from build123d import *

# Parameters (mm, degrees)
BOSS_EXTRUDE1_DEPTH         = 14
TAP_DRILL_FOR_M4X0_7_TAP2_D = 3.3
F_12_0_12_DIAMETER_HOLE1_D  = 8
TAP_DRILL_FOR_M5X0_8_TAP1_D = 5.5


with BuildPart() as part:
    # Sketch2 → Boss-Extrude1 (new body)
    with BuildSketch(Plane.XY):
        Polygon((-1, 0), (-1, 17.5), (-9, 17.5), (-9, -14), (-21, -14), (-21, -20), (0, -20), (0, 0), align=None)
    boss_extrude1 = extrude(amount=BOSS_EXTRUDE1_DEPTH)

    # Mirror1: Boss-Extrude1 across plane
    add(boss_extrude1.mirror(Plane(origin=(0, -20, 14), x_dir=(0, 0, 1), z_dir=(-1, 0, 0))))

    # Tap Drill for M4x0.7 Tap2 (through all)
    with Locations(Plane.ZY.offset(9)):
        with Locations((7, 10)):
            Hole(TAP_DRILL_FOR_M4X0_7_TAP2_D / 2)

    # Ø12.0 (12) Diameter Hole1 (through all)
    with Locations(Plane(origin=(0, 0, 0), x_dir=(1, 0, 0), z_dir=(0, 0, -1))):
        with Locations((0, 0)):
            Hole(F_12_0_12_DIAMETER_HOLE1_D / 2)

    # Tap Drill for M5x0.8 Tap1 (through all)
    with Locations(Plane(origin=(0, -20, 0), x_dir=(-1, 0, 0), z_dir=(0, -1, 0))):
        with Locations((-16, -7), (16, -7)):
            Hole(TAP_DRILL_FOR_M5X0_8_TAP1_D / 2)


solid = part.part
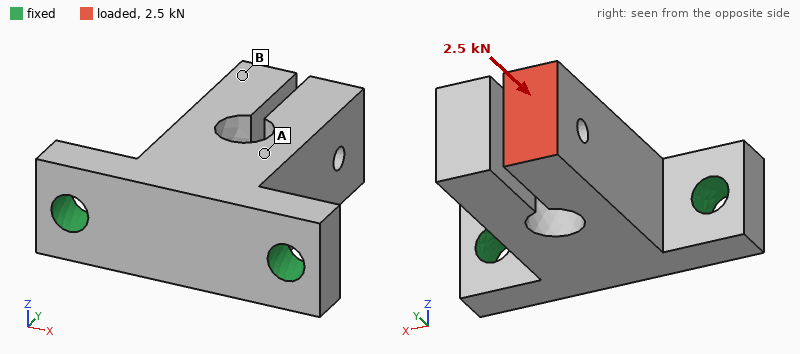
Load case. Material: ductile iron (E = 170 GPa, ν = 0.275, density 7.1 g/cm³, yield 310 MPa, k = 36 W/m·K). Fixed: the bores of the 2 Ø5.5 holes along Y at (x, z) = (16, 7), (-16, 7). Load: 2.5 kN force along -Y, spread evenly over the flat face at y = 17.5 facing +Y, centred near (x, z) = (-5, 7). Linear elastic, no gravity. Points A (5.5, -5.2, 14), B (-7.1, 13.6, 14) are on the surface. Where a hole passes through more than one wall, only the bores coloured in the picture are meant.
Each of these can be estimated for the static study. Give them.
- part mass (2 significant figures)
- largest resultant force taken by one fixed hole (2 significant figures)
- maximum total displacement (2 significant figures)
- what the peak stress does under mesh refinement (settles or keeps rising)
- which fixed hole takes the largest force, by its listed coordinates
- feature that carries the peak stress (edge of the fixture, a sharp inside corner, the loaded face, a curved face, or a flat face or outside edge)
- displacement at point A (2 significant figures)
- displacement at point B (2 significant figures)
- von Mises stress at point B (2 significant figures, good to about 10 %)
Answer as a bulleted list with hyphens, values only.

- 71 g
- 1.8 kN
- 16 µm
- keeps rising
- (-16, 7)
- edge of the fixture
- 3.2 µm
- 10 µm
- 22 MPa
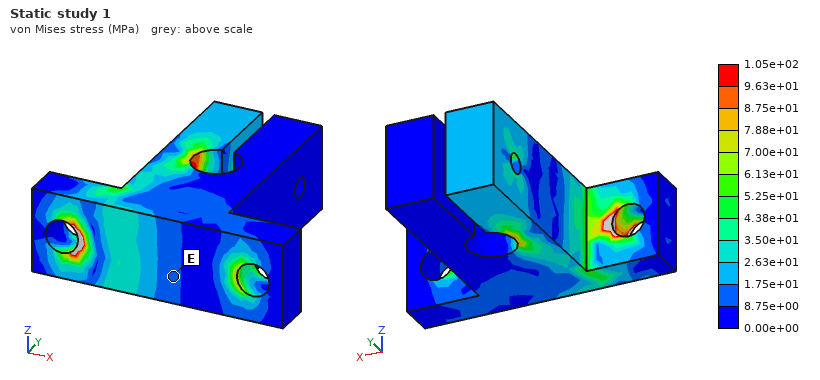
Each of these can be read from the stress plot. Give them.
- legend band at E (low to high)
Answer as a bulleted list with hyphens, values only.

- 8.75e+00 to 1.75e+01 MPa
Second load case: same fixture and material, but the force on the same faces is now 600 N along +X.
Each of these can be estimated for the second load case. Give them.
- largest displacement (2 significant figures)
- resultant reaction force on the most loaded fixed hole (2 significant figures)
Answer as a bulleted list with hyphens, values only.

- 86 µm
- 980 N
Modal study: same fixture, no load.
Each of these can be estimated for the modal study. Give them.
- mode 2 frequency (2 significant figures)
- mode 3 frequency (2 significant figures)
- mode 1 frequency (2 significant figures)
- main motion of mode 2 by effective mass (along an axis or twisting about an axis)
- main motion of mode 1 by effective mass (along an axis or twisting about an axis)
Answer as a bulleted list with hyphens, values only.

- 5600 Hz
- 6400 Hz
- 4000 Hz
- along X
- along Z
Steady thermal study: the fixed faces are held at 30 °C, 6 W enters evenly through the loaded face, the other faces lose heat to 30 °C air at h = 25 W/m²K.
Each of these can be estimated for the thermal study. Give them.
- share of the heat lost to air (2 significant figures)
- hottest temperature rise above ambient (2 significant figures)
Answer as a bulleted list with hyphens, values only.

- 23 %
- 53 K
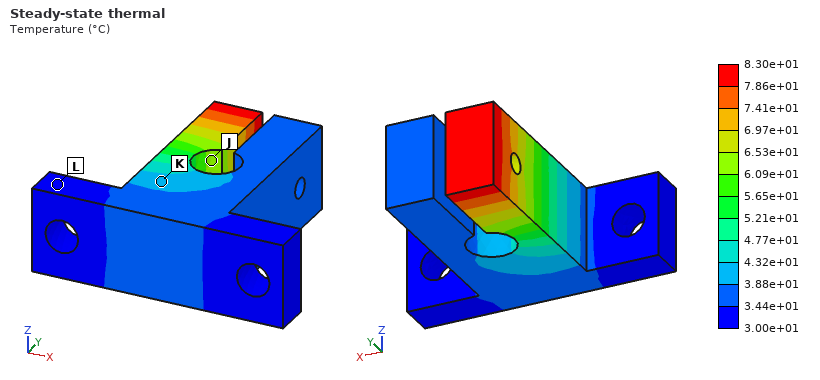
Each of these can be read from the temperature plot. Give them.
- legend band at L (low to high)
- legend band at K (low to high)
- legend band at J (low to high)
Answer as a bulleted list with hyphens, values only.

- 3.00e+01 to 3.44e+01 °C
- 3.88e+01 to 4.32e+01 °C
- 6.09e+01 to 6.53e+01 °C
